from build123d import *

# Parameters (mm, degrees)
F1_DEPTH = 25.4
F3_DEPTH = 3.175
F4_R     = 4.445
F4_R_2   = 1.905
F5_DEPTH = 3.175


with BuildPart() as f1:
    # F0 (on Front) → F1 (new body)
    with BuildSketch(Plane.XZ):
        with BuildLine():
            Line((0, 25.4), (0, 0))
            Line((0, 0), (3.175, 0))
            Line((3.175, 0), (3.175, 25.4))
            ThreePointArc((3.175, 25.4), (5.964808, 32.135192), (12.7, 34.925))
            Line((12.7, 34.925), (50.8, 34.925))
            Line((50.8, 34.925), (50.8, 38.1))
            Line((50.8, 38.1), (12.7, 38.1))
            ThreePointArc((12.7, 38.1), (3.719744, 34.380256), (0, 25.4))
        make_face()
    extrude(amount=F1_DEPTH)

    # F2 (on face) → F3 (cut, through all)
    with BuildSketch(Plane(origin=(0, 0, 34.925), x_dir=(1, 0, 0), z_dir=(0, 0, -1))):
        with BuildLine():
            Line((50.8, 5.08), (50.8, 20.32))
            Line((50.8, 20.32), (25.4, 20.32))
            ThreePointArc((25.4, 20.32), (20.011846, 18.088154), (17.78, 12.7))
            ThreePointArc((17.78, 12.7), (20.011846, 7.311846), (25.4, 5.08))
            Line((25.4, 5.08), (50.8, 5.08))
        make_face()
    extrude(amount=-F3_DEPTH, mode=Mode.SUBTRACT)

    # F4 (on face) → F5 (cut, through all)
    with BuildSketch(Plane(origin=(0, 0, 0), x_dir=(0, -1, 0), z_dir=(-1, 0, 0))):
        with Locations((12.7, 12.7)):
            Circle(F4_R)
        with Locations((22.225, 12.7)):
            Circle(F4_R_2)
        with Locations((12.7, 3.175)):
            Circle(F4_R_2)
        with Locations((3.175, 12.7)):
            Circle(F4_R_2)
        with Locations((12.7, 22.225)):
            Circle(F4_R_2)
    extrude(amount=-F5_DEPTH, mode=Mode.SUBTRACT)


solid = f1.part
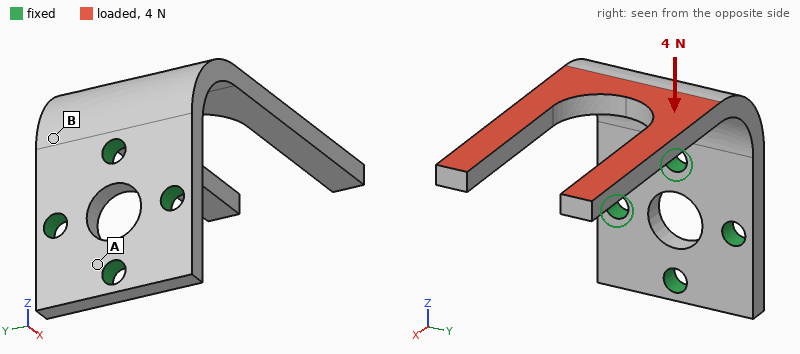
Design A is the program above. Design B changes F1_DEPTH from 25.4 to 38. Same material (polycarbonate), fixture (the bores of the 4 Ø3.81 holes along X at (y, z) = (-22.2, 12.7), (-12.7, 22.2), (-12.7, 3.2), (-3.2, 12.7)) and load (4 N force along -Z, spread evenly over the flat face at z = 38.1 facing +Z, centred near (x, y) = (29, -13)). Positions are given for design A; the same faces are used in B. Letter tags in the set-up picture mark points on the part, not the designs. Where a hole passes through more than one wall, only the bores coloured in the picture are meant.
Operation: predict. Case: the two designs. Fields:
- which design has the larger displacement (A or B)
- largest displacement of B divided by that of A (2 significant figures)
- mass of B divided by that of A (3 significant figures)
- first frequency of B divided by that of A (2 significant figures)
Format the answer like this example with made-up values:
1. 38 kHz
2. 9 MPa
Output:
1. A
2. 0.78
3. 1.69
4. 0.80
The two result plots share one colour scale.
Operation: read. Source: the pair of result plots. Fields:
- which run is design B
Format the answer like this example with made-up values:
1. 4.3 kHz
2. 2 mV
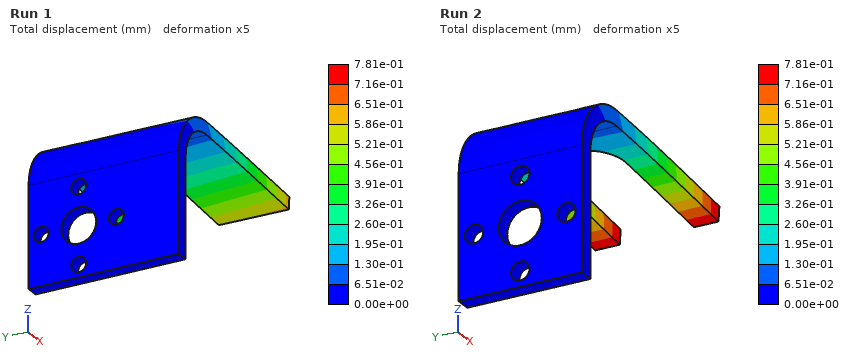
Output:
1. Run 1
